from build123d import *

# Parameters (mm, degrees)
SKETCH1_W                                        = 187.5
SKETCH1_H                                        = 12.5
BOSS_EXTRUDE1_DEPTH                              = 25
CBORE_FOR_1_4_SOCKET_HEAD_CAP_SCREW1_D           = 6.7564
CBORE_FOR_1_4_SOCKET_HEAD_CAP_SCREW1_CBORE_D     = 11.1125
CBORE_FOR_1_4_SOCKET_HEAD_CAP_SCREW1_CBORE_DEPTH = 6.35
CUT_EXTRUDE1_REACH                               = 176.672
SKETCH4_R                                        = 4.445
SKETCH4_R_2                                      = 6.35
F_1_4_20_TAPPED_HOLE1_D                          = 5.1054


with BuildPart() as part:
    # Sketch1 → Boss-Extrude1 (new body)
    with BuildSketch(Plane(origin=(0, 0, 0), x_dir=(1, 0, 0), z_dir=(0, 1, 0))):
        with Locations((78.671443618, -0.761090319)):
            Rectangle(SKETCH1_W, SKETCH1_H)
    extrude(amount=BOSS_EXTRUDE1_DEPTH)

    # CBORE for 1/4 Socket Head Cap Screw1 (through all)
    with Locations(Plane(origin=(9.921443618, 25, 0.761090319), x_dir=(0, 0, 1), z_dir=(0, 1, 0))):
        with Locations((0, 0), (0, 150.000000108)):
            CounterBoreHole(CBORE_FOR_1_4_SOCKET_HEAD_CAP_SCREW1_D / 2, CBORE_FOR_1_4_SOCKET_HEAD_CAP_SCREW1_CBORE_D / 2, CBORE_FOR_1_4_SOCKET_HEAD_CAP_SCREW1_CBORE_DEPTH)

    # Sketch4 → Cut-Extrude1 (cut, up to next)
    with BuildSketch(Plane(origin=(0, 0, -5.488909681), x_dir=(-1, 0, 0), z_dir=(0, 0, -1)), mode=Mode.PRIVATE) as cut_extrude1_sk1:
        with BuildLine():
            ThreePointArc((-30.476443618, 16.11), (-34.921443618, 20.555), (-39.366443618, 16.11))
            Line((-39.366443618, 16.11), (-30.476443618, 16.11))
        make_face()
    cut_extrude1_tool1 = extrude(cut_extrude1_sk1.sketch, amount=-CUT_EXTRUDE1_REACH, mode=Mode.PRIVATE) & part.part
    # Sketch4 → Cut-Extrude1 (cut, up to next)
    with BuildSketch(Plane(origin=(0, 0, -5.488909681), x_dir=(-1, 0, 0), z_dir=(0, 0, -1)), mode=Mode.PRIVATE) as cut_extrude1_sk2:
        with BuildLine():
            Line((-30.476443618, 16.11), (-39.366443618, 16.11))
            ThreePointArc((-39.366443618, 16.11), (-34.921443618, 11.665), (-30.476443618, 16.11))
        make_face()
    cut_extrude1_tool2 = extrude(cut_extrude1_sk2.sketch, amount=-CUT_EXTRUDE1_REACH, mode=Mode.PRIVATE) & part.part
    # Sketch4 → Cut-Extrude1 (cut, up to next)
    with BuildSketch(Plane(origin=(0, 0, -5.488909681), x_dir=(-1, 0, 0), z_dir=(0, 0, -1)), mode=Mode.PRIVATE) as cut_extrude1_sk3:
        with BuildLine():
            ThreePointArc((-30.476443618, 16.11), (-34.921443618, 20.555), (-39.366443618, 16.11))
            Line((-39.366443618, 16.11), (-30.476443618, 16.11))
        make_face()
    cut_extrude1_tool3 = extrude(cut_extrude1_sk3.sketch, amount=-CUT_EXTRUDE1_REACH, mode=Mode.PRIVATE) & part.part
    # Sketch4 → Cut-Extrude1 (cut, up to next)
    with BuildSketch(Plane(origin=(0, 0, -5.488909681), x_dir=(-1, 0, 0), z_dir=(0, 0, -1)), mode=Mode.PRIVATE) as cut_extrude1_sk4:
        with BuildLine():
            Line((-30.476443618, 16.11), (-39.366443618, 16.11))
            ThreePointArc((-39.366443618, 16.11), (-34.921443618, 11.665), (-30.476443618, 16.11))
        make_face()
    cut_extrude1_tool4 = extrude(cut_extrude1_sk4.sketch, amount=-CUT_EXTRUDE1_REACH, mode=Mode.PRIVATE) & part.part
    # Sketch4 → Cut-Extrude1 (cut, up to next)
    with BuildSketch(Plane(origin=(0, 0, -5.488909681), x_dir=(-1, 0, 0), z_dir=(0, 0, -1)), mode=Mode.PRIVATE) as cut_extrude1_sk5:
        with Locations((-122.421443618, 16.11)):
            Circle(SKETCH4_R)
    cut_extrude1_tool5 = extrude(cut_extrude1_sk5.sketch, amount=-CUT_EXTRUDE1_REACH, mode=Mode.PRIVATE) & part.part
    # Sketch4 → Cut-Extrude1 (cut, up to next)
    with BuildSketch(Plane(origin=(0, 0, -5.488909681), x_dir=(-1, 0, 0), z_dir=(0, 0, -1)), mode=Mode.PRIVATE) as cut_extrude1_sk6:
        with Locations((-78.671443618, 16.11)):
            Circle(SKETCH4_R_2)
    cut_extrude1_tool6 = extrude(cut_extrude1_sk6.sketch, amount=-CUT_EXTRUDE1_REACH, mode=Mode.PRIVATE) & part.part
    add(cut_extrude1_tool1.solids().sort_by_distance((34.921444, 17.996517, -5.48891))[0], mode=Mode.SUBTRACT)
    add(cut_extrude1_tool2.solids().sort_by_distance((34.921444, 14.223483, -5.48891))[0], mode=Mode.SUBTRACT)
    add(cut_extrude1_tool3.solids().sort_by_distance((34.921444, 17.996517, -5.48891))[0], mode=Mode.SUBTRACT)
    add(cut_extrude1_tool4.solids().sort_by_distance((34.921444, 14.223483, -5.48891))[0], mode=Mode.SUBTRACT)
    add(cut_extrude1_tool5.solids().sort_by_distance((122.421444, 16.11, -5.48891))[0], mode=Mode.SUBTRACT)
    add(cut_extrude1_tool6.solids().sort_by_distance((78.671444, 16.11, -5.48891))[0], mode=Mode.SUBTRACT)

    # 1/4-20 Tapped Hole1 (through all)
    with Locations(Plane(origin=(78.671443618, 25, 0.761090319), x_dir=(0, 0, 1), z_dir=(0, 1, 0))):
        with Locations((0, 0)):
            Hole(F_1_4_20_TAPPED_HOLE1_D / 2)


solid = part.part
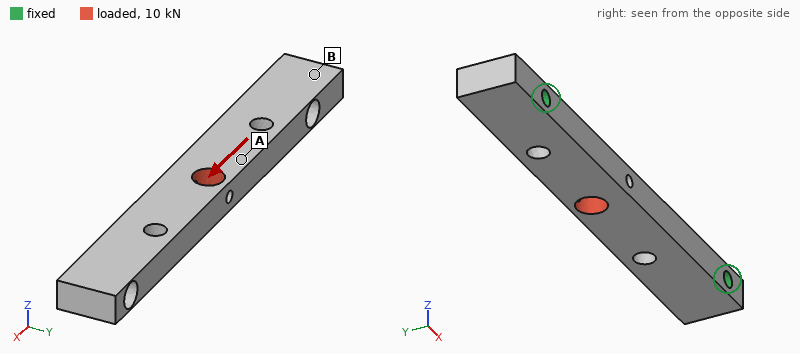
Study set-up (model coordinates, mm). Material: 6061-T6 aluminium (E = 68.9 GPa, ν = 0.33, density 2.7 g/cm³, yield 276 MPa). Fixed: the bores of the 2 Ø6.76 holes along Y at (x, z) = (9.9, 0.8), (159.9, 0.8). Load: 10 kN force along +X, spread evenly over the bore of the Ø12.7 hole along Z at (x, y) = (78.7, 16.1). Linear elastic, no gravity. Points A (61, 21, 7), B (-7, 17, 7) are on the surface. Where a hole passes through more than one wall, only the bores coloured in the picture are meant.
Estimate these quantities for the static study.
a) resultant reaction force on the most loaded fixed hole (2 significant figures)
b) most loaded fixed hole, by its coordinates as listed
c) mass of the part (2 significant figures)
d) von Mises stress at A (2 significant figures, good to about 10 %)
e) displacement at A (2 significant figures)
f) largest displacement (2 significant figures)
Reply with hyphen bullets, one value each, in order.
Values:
- 5.3 kN
- (9.9, 0.8)
- 140 g
- 21 MPa
- 17 µm
- 23 µm
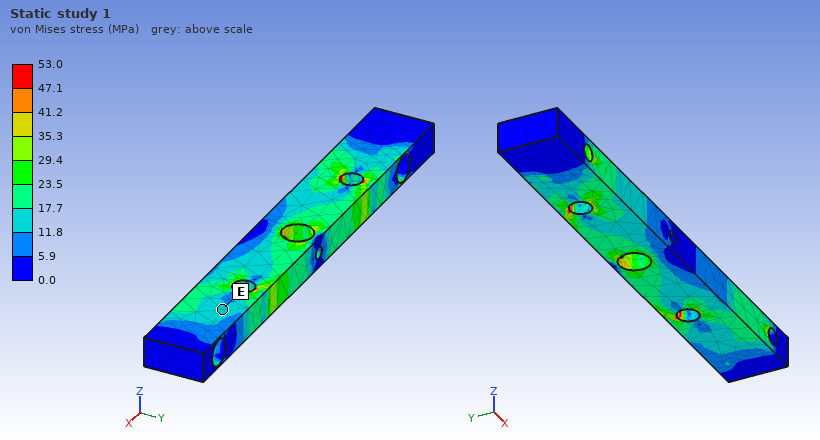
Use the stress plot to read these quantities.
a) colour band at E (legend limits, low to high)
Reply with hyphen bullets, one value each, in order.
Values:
- 11.8 to 17.7 MPa
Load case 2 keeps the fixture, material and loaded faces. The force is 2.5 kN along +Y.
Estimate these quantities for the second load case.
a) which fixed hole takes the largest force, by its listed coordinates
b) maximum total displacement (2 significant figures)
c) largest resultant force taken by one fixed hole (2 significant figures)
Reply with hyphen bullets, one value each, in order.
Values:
- (9.9, 0.8)
- 73 µm
- 1.4 kN
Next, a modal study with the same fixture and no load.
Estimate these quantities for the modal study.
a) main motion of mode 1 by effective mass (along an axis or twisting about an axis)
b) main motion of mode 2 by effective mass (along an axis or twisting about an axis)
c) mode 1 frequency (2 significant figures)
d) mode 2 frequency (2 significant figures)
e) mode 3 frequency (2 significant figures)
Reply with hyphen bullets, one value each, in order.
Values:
- along Z
- along Y
- 2600 Hz
- 4400 Hz
- 6800 Hz
